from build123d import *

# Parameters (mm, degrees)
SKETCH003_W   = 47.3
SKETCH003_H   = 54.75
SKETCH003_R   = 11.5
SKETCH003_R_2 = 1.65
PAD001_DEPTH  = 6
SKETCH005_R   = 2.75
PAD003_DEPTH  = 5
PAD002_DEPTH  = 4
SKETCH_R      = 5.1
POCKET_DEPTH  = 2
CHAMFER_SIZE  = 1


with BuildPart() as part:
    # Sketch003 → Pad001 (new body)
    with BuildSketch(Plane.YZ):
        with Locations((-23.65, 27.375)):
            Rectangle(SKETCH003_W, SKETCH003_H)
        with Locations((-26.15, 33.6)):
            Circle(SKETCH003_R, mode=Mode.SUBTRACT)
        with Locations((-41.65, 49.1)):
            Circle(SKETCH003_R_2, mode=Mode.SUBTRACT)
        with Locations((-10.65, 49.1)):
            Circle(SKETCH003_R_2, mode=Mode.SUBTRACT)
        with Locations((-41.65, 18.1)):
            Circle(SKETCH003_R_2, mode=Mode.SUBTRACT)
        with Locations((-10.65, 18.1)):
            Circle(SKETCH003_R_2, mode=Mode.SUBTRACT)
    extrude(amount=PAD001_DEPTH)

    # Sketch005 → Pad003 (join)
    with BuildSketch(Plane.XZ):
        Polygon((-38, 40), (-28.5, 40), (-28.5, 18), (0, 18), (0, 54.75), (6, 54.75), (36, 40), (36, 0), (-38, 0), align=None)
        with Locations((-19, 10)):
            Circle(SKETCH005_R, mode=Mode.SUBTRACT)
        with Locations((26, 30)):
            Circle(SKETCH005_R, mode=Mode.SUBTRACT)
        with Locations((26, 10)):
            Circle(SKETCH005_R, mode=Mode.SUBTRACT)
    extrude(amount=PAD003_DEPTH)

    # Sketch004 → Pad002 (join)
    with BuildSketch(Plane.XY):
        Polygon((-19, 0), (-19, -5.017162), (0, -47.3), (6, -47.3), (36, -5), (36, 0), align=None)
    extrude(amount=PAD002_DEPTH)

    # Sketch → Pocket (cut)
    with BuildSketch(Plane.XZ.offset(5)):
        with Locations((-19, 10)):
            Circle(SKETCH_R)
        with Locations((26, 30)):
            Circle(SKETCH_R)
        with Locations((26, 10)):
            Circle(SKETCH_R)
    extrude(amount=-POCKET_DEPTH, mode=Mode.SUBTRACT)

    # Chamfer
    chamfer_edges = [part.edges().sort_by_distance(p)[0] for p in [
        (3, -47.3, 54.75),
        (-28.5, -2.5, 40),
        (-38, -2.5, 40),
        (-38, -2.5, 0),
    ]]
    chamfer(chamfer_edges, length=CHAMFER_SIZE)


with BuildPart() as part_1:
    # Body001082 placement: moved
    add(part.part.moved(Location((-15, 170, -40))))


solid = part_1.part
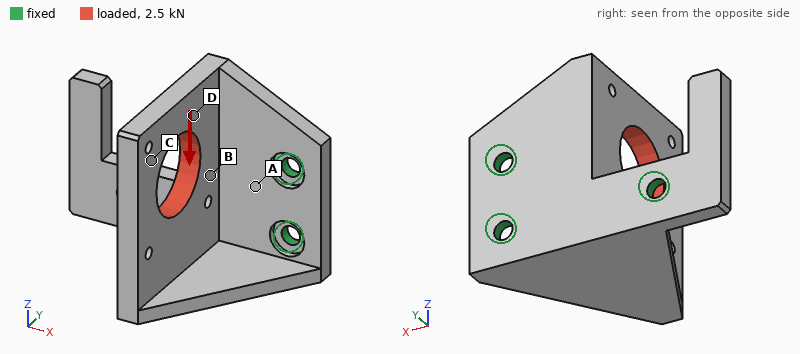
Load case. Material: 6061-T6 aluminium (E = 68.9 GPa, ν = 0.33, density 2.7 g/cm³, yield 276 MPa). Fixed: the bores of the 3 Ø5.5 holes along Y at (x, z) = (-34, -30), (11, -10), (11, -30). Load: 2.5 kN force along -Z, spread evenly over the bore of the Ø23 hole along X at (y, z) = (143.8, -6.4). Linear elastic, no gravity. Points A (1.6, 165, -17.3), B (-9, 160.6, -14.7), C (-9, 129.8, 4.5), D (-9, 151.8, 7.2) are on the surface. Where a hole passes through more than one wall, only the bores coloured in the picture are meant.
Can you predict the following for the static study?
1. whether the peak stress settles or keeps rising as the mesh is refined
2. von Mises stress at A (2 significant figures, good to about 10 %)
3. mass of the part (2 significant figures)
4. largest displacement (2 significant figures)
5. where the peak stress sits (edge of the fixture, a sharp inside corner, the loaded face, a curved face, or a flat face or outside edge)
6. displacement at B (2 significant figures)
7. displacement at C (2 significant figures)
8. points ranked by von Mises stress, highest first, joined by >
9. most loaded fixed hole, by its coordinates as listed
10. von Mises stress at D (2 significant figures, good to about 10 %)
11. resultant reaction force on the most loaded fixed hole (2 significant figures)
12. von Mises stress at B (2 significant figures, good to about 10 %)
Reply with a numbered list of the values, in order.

1. keeps rising
2. 120 MPa
3. 75 g
4. 0.53 mm
5. edge of the fixture
6. 0.13 mm
7. 0.43 mm
8. A > B > D > C
9. (11, -10)
10. 49 MPa
11. 3.2 kN
12. 86 MPa
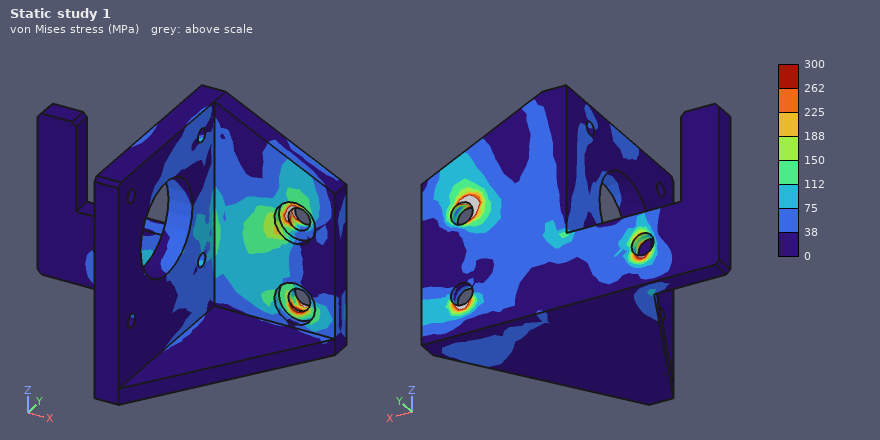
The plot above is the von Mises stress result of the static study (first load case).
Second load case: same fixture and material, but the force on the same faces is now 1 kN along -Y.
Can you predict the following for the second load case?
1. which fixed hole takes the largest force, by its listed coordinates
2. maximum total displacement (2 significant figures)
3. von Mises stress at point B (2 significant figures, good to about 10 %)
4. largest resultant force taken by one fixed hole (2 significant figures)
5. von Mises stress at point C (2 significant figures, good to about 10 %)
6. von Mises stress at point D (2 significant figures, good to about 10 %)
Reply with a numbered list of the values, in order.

1. (11, -10)
2. 0.24 mm
3. 31 MPa
4. 930 N
5. 11 MPa
6. 25 MPa
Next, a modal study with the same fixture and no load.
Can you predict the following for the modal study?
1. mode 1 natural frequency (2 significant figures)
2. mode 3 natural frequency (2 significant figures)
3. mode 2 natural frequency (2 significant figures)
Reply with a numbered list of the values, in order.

1. 1800 Hz
2. 3400 Hz
3. 2900 Hz
